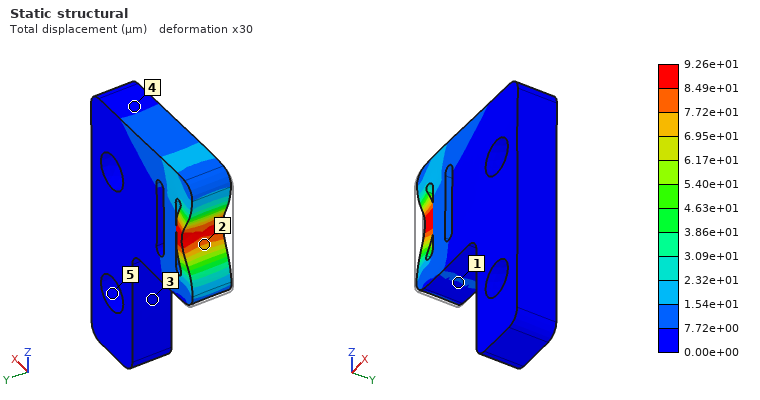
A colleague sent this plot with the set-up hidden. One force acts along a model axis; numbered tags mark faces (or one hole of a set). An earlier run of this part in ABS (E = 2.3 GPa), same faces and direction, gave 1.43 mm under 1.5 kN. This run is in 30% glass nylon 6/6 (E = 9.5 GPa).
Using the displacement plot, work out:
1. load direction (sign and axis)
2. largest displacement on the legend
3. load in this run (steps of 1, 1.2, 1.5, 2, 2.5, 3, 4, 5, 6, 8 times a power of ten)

+X
9.26e+01 µm
400 N
